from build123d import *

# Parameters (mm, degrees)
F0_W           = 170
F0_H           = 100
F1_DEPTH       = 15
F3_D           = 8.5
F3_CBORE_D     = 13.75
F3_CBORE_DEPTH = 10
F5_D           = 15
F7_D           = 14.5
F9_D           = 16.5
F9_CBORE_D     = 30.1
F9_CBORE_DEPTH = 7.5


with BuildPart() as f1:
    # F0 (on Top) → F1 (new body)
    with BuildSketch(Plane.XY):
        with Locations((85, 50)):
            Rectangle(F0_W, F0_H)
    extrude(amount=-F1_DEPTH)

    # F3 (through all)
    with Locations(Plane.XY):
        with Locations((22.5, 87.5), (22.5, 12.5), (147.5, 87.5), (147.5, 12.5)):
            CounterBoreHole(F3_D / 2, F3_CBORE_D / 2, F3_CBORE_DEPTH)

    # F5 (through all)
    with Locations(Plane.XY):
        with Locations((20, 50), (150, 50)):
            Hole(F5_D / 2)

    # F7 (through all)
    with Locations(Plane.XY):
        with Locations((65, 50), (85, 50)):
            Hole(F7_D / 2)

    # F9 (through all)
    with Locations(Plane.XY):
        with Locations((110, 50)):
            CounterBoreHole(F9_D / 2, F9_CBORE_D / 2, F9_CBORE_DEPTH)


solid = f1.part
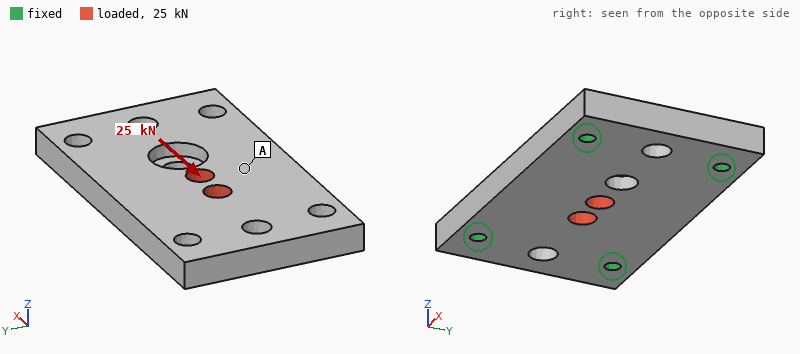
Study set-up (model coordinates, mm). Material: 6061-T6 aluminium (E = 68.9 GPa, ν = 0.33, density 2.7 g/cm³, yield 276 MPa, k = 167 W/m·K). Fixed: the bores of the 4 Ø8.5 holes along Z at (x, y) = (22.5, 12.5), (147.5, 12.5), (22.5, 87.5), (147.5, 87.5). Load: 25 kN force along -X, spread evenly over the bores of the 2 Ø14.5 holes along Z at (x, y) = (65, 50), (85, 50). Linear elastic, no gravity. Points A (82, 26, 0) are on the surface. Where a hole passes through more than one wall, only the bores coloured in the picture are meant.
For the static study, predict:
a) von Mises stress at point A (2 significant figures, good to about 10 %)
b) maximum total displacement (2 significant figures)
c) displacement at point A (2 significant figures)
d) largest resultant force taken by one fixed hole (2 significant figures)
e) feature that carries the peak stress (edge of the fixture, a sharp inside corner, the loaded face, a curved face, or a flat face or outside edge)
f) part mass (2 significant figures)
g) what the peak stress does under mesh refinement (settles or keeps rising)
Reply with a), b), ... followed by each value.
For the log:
a) 9.6 MPa
b) 34 µm
c) 14 µm
d) 6.9 kN
e) edge of the fixture
f) 620 g
g) keeps rising
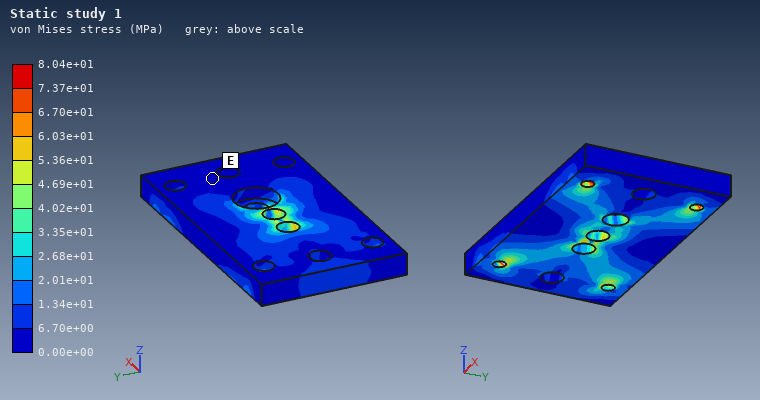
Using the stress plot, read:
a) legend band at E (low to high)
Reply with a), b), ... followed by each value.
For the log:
a) 0.00e+00 to 6.70e+00 MPa
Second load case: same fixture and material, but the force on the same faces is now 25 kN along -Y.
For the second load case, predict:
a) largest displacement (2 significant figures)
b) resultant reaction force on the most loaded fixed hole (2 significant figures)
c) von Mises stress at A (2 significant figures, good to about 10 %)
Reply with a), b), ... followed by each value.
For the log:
a) 40 µm
b) 8.8 kN
c) 11 MPa
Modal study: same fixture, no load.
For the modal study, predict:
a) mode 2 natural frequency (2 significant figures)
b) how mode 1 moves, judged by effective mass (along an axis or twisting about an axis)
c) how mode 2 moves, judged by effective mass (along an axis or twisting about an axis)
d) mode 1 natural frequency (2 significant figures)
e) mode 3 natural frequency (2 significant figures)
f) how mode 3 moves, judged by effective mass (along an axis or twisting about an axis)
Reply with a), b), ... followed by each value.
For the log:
a) 4700 Hz
b) along Z
c) twisting about X
d) 3000 Hz
e) 6800 Hz
f) along Z
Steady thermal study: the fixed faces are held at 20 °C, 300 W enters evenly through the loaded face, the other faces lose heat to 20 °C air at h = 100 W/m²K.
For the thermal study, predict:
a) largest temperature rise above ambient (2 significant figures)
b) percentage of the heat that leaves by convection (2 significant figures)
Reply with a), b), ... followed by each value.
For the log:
a) 63 K
b) 28 %
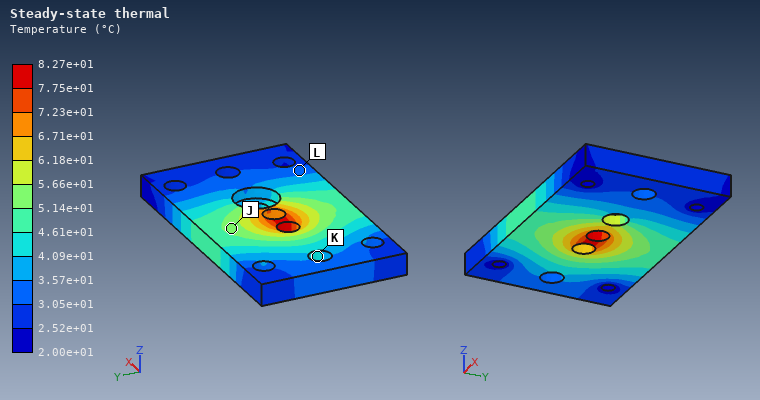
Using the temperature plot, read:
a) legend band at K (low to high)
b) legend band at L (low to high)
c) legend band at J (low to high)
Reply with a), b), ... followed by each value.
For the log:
a) 4.09e+01 to 4.61e+01 °C
b) 3.05e+01 to 3.57e+01 °C
c) 5.14e+01 to 5.66e+01 °C
